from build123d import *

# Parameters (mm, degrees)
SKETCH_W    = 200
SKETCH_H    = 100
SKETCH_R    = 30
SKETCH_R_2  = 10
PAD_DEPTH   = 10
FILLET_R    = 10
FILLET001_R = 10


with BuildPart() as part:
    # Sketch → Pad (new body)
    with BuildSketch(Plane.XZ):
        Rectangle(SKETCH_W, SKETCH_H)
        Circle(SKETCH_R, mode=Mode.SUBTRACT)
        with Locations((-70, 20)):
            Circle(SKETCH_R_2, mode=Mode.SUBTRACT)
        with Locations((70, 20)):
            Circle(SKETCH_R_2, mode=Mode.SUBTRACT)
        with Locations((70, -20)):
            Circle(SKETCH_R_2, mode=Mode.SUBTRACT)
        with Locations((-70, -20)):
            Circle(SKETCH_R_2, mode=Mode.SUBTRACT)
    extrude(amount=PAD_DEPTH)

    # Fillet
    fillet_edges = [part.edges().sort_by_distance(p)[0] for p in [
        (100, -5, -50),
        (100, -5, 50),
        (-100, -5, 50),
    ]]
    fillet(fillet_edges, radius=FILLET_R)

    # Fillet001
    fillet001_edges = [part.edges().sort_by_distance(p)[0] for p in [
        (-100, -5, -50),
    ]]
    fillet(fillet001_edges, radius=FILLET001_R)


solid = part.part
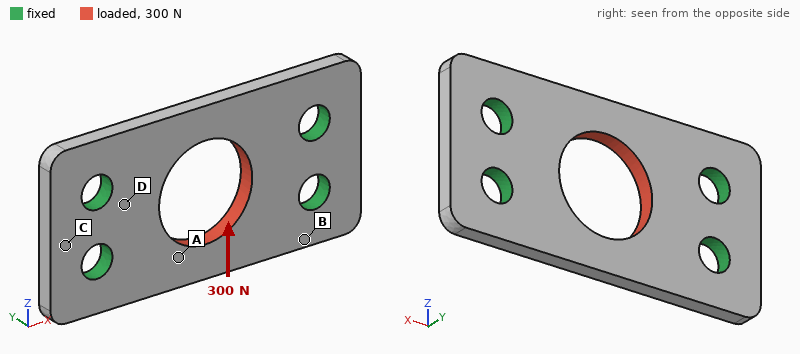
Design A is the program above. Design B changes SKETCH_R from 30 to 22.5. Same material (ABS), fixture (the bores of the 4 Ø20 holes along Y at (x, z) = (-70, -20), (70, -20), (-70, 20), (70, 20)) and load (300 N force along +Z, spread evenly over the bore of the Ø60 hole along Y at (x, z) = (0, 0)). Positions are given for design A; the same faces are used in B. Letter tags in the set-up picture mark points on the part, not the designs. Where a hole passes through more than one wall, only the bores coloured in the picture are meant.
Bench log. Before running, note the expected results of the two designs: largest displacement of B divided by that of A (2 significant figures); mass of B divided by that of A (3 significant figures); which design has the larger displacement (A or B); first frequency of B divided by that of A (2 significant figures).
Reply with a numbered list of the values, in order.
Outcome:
1. 0.91
2. 1.08
3. A
4. 0.95
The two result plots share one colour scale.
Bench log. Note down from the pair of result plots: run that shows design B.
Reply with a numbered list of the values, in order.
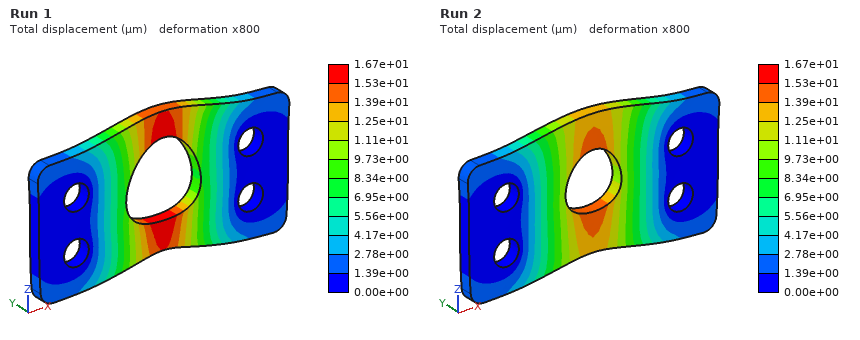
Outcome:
1. Run 2
